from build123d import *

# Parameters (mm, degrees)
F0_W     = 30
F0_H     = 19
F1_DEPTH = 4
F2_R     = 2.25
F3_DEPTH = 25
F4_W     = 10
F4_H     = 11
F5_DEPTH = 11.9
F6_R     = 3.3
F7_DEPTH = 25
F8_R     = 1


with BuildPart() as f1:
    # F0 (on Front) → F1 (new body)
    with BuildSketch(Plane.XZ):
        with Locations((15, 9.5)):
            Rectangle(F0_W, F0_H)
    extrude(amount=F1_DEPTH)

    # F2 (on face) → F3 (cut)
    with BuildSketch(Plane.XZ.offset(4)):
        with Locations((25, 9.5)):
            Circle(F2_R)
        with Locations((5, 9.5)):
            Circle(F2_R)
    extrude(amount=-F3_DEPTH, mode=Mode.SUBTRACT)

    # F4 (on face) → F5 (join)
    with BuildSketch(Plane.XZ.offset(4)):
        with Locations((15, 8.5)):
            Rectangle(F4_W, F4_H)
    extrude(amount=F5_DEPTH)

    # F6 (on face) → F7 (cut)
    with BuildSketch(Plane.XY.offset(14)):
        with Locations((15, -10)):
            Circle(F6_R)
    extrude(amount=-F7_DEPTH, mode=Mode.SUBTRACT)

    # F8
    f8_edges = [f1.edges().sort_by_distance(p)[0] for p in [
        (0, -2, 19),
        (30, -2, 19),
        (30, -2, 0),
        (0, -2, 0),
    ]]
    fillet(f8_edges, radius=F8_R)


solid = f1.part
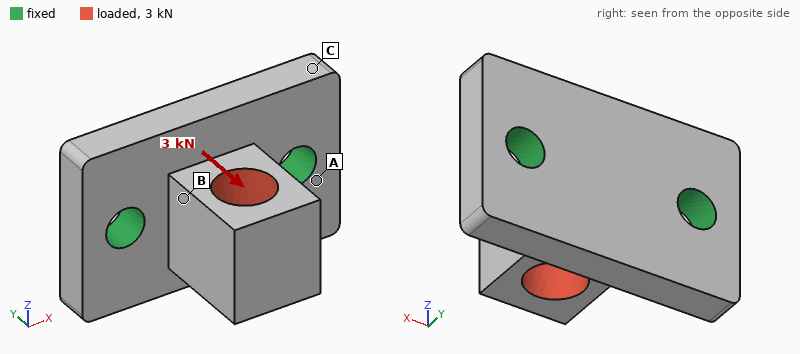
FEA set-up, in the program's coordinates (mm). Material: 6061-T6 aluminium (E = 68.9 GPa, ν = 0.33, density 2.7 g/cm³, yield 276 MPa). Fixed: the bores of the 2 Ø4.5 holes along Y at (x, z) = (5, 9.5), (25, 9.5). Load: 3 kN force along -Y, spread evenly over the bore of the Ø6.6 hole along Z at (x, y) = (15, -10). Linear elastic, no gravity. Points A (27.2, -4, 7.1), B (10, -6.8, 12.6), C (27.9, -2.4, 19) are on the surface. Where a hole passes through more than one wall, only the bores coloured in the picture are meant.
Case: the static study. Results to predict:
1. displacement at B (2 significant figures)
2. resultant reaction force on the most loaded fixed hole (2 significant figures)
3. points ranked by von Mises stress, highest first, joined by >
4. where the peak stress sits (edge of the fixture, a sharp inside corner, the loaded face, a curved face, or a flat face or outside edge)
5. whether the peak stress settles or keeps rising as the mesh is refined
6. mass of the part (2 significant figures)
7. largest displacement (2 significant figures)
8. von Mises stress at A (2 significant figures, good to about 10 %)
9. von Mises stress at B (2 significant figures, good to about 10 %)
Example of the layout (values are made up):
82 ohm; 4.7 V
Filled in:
12 µm; 1.5 kN; B > A > C; edge of the fixture; keeps rising; 8.3 g; 26 µm; 34 MPa; 56 MPa
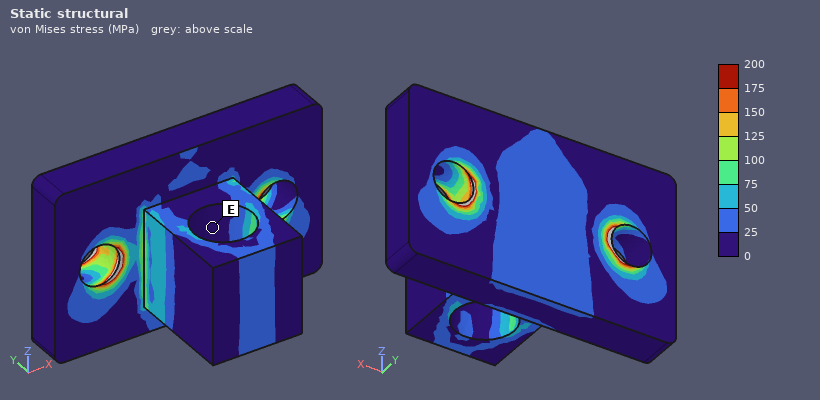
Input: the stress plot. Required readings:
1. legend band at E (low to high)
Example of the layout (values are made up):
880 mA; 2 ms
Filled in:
0 to 25 MPa
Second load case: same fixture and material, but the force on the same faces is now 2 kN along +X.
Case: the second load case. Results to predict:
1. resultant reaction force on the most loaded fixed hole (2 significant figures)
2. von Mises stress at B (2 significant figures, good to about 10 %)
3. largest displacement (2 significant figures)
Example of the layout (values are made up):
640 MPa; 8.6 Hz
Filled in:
1.5 kN; 120 MPa; 53 µm
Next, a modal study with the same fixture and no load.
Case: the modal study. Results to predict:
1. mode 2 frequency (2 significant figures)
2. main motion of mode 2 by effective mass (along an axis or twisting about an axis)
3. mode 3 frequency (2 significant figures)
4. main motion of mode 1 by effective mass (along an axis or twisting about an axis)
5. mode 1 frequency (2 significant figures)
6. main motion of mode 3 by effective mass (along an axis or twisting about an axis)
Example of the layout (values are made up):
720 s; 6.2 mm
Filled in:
22 kHz; along X; 32 kHz; along Z; 16 kHz; along Y
